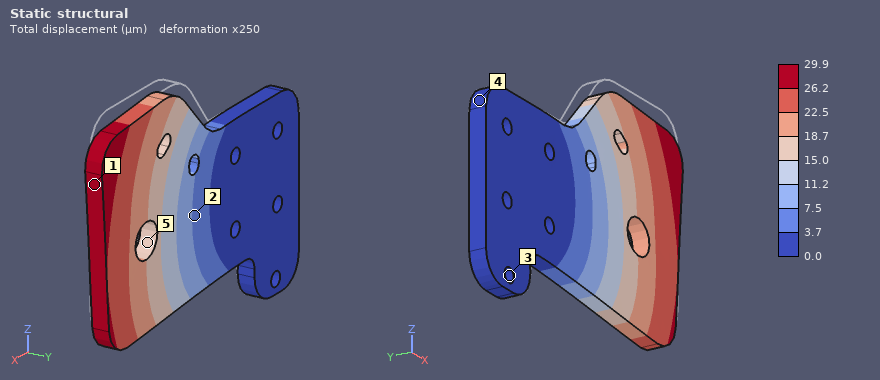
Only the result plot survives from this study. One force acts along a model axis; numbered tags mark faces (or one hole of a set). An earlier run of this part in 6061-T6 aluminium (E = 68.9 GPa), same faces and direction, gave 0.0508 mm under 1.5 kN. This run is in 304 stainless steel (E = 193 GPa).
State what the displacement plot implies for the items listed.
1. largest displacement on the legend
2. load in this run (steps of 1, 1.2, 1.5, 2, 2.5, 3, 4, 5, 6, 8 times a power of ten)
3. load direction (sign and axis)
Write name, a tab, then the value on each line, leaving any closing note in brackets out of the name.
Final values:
largest displacement on the legend	29.9 µm
load in this run	2.5 kN
load direction	-Z
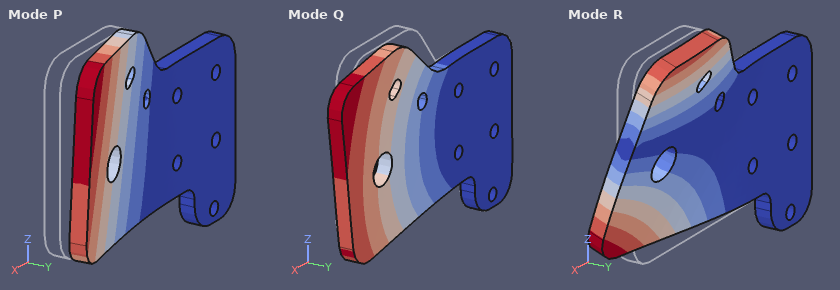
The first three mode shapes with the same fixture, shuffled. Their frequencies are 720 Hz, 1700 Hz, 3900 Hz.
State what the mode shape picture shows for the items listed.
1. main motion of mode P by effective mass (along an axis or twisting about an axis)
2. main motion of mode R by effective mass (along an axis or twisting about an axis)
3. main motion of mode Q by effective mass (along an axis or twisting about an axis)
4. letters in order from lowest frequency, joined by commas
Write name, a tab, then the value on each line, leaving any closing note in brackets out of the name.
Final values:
main motion of mode P by effective mass	along Y
main motion of mode R by effective mass	twisting about X
main motion of mode Q by effective mass	along Z
letters in order from lowest frequency, joined by commas	P, R, Q
